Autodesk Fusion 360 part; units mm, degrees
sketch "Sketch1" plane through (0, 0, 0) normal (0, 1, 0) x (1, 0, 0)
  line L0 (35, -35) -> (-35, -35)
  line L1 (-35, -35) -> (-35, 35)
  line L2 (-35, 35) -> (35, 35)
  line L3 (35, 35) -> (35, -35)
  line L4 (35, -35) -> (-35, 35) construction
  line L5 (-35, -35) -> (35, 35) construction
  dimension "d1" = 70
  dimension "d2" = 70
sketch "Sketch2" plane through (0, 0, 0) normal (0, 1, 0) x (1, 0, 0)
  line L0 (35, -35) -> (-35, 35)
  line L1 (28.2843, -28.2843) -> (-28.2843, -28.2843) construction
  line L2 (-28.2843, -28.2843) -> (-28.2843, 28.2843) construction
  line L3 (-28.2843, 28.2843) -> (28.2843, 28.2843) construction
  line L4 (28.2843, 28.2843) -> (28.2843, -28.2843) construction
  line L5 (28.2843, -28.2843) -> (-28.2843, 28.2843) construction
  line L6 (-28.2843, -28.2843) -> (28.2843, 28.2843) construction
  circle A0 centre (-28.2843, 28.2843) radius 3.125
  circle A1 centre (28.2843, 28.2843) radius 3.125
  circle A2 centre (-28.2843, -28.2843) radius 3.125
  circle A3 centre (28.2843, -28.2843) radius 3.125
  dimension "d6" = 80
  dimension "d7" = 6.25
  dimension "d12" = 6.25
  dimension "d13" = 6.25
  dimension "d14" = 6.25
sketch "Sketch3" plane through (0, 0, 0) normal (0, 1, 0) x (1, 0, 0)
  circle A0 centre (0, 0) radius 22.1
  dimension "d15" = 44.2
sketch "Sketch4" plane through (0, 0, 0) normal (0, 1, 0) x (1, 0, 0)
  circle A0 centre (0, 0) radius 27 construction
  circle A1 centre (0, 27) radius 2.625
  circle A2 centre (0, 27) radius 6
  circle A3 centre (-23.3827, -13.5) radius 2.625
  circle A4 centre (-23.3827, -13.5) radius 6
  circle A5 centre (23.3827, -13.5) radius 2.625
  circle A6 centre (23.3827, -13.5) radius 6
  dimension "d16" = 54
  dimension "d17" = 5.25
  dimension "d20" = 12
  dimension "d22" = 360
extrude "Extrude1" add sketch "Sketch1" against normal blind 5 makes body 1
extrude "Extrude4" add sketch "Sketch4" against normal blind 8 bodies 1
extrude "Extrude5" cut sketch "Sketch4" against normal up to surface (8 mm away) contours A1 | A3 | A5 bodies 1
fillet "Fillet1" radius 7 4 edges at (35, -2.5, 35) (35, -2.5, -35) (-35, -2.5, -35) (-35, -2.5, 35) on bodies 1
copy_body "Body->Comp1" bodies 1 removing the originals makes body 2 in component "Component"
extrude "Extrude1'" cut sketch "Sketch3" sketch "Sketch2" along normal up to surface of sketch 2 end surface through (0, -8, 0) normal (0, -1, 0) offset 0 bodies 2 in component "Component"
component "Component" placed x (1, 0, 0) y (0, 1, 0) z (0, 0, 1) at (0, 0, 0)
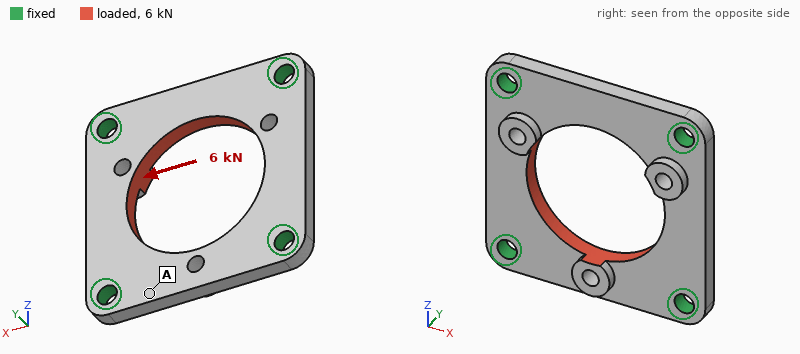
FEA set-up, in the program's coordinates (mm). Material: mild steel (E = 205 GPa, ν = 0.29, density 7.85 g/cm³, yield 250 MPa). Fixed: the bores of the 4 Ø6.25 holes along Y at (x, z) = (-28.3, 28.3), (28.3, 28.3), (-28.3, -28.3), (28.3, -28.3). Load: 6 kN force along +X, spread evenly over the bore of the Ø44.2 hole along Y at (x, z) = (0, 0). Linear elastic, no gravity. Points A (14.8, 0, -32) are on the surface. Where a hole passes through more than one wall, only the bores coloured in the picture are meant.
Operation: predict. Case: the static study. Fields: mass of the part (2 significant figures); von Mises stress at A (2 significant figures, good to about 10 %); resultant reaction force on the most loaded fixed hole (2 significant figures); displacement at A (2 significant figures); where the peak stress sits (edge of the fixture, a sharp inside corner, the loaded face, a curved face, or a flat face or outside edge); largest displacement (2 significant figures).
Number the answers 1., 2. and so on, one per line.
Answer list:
1. 130 g
2. 13 MPa
3. 1.5 kN
4. 1.2 µm
5. edge of the fixture
6. 5.4 µm
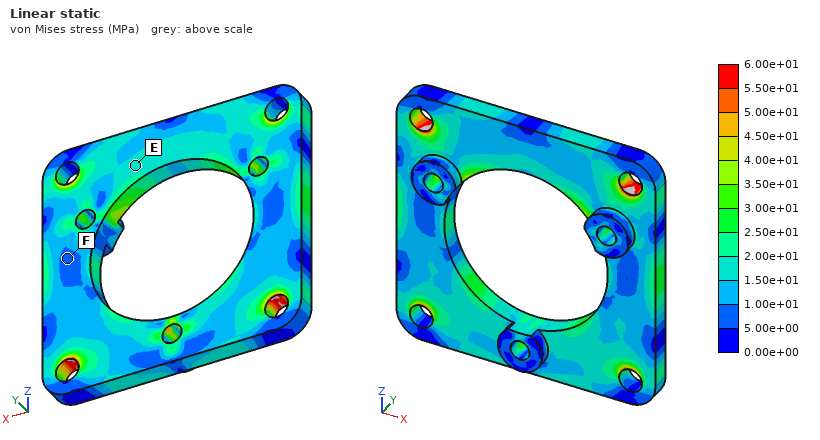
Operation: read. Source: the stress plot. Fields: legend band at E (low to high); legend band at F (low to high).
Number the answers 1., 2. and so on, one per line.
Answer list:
1. 1.50e+01 to 2.00e+01 MPa
2. 5.00e+00 to 1.00e+01 MPa
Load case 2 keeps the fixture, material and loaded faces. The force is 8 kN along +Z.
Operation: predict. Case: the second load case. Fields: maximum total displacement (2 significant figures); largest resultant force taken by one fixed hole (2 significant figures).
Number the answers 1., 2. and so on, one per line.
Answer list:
1. 8.7 µm
2. 2.0 kN
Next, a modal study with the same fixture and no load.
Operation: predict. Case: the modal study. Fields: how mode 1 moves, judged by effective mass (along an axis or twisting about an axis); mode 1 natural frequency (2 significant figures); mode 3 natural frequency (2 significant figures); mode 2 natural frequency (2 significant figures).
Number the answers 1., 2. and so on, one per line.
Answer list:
1. along Y
2. 8900 Hz
3. 9300 Hz
4. 9300 Hz
